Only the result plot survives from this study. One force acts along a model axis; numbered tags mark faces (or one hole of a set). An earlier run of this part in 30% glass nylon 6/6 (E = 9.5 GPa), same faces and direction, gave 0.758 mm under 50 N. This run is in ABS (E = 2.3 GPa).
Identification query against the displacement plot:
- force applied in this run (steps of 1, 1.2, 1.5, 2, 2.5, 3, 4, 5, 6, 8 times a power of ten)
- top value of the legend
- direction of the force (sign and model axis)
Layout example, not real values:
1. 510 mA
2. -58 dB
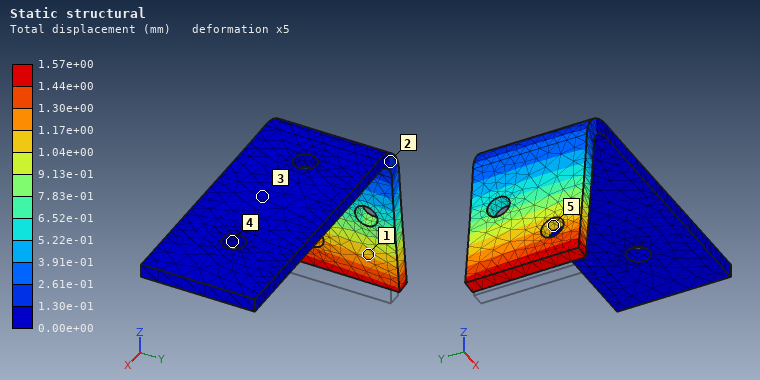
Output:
1. 25 N
2. 1.57e+00 mm
3. -X
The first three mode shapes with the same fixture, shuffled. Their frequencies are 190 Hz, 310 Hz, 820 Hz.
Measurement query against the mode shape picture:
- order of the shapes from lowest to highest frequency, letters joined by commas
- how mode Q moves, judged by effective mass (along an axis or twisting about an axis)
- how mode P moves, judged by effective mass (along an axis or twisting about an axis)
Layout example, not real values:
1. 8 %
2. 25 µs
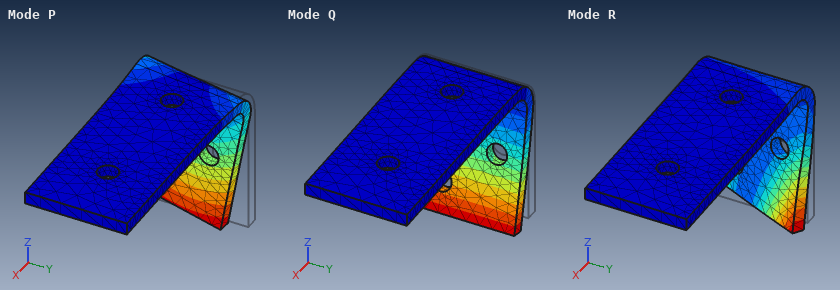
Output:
1. Q, P, R
2. along X
3. along Y
